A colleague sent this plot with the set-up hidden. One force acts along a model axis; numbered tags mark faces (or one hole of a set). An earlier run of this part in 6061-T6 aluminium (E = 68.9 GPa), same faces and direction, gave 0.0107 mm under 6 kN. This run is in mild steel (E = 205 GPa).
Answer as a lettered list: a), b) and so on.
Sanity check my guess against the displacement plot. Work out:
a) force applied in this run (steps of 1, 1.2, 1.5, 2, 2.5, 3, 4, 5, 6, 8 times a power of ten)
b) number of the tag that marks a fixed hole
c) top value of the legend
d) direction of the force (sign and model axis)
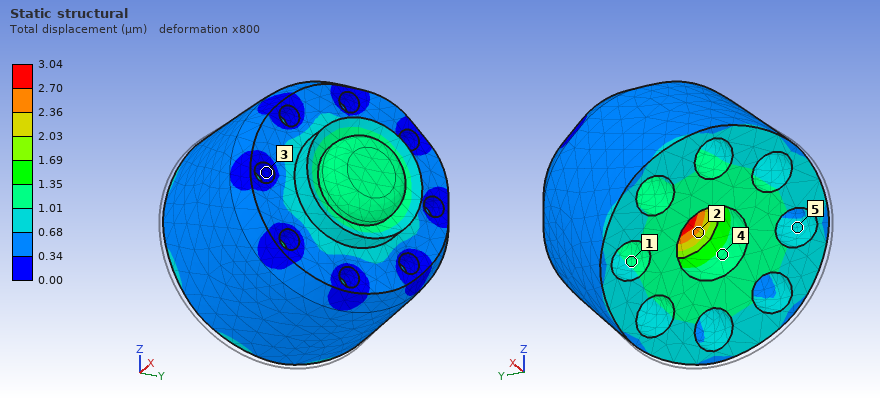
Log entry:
a) 5 kN
b) 3
c) 3.04 µm
d) +X
